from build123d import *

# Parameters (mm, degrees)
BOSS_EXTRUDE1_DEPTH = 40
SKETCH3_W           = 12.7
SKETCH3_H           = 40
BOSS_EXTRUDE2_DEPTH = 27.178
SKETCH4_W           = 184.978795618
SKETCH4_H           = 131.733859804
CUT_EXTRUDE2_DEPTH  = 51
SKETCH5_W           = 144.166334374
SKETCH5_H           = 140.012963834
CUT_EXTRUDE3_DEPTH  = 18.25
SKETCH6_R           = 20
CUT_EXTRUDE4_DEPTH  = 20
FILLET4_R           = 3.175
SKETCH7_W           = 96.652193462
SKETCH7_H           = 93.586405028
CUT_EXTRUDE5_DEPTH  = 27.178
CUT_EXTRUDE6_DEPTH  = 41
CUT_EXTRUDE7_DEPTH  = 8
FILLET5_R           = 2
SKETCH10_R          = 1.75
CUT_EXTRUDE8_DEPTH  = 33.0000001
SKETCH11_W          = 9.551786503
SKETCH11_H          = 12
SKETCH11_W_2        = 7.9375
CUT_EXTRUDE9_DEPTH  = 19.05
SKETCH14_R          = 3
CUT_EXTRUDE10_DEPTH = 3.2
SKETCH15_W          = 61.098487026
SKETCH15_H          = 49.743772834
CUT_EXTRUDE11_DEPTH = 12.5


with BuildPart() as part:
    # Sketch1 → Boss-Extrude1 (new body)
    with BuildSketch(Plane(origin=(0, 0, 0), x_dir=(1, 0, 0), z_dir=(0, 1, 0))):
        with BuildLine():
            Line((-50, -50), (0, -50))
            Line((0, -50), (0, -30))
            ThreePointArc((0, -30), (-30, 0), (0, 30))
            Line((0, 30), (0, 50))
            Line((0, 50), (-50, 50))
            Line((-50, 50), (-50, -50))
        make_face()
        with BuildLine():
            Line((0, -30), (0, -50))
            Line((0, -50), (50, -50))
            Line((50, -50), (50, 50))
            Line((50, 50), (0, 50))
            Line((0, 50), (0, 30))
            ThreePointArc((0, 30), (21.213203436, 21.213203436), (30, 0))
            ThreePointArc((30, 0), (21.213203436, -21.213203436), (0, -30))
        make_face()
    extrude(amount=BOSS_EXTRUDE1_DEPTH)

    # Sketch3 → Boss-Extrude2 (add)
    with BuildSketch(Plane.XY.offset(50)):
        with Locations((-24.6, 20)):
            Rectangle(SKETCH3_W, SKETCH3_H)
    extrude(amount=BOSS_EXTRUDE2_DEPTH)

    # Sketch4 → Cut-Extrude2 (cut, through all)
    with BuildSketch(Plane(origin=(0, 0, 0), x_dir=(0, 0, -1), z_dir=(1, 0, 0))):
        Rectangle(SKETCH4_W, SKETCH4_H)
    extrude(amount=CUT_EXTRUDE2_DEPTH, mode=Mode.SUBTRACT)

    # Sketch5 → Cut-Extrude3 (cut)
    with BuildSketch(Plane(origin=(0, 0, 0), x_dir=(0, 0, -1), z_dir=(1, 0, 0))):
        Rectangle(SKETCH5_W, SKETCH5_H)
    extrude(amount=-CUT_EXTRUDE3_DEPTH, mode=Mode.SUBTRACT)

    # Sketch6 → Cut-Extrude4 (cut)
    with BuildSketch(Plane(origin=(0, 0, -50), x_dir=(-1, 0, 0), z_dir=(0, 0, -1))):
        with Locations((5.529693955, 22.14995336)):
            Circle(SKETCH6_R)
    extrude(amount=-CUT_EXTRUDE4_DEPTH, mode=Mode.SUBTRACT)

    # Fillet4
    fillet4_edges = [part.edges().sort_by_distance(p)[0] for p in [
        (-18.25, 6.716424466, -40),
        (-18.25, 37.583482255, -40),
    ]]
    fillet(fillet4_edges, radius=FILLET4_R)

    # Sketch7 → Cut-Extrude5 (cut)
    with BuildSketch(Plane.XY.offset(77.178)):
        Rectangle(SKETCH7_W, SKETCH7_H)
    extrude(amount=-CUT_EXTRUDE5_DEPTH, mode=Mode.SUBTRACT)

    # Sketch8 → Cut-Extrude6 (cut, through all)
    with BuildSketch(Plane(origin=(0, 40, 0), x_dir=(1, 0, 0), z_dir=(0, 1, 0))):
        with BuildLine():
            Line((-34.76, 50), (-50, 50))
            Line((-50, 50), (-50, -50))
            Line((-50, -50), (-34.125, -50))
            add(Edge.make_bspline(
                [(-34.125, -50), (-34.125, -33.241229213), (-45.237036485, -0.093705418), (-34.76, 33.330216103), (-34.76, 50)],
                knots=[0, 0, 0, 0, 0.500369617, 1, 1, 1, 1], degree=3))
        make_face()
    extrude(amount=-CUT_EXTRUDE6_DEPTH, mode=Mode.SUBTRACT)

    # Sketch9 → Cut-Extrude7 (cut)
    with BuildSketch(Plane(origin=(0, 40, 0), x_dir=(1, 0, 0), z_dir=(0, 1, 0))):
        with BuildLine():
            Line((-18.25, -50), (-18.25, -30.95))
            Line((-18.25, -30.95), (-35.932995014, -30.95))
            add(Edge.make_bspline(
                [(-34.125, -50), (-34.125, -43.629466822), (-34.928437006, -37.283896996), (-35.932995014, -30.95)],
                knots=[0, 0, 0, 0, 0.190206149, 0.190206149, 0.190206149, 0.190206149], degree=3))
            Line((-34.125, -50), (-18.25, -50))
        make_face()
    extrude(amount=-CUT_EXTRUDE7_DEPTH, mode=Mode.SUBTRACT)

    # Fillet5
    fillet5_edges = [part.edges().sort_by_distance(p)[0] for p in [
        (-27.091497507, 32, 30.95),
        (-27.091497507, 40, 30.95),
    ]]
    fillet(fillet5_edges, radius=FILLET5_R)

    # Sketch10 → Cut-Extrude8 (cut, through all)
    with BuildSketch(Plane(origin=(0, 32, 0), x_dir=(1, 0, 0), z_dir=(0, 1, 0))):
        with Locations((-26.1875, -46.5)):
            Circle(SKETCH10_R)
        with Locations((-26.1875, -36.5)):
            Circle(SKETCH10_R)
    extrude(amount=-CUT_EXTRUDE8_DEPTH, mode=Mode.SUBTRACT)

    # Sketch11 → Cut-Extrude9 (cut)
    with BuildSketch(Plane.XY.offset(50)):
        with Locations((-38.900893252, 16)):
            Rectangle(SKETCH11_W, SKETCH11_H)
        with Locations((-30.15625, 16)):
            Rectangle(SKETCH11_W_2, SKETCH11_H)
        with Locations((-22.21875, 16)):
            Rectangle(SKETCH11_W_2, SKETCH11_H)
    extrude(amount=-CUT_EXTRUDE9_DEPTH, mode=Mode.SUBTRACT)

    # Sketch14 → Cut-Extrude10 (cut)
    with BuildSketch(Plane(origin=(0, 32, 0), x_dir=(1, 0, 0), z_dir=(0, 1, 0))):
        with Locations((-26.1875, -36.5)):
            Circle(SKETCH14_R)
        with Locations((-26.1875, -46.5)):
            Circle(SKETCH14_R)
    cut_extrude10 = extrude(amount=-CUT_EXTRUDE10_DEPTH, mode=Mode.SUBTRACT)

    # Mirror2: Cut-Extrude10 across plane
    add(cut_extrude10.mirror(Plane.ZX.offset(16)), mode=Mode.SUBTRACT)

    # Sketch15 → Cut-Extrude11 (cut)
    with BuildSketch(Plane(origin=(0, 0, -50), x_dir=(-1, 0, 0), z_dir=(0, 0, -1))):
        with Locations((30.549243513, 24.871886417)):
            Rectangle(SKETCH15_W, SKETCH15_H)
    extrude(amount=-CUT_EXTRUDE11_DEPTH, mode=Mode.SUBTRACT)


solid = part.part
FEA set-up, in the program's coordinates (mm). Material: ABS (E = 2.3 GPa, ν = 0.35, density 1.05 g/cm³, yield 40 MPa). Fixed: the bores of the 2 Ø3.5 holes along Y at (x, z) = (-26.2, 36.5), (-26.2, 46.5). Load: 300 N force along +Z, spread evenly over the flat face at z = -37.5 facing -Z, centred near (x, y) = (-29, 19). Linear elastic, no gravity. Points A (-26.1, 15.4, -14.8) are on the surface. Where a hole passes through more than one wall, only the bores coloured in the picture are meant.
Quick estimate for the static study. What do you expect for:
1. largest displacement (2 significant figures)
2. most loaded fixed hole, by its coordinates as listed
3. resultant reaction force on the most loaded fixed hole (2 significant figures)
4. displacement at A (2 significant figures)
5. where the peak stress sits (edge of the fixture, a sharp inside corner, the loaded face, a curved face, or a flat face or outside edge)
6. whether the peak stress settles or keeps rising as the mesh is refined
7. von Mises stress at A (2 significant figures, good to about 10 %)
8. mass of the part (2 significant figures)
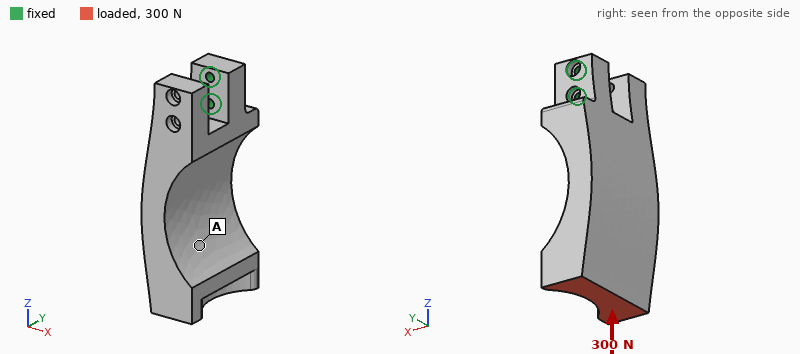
0.73 mm
(-26.2, 36.5)
300 N
0.45 mm
edge of the fixture
keeps rising
1.6 MPa
46 g
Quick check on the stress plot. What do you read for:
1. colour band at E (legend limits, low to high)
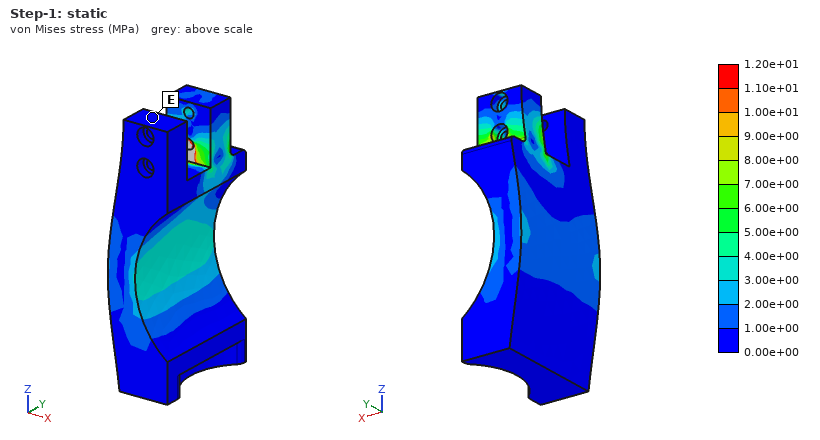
0.00e+00 to 1.00e+00 MPa
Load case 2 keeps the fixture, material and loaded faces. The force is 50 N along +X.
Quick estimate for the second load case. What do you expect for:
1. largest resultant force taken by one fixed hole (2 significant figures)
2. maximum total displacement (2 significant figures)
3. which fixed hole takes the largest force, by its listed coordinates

300 N
1.00 mm
(-26.2, 36.5)
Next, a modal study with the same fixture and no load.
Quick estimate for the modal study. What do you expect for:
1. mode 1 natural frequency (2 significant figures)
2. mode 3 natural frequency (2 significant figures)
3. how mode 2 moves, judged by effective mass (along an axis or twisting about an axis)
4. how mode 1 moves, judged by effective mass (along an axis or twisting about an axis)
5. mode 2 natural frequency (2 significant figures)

270 Hz
810 Hz
along X
along Y
330 Hz
